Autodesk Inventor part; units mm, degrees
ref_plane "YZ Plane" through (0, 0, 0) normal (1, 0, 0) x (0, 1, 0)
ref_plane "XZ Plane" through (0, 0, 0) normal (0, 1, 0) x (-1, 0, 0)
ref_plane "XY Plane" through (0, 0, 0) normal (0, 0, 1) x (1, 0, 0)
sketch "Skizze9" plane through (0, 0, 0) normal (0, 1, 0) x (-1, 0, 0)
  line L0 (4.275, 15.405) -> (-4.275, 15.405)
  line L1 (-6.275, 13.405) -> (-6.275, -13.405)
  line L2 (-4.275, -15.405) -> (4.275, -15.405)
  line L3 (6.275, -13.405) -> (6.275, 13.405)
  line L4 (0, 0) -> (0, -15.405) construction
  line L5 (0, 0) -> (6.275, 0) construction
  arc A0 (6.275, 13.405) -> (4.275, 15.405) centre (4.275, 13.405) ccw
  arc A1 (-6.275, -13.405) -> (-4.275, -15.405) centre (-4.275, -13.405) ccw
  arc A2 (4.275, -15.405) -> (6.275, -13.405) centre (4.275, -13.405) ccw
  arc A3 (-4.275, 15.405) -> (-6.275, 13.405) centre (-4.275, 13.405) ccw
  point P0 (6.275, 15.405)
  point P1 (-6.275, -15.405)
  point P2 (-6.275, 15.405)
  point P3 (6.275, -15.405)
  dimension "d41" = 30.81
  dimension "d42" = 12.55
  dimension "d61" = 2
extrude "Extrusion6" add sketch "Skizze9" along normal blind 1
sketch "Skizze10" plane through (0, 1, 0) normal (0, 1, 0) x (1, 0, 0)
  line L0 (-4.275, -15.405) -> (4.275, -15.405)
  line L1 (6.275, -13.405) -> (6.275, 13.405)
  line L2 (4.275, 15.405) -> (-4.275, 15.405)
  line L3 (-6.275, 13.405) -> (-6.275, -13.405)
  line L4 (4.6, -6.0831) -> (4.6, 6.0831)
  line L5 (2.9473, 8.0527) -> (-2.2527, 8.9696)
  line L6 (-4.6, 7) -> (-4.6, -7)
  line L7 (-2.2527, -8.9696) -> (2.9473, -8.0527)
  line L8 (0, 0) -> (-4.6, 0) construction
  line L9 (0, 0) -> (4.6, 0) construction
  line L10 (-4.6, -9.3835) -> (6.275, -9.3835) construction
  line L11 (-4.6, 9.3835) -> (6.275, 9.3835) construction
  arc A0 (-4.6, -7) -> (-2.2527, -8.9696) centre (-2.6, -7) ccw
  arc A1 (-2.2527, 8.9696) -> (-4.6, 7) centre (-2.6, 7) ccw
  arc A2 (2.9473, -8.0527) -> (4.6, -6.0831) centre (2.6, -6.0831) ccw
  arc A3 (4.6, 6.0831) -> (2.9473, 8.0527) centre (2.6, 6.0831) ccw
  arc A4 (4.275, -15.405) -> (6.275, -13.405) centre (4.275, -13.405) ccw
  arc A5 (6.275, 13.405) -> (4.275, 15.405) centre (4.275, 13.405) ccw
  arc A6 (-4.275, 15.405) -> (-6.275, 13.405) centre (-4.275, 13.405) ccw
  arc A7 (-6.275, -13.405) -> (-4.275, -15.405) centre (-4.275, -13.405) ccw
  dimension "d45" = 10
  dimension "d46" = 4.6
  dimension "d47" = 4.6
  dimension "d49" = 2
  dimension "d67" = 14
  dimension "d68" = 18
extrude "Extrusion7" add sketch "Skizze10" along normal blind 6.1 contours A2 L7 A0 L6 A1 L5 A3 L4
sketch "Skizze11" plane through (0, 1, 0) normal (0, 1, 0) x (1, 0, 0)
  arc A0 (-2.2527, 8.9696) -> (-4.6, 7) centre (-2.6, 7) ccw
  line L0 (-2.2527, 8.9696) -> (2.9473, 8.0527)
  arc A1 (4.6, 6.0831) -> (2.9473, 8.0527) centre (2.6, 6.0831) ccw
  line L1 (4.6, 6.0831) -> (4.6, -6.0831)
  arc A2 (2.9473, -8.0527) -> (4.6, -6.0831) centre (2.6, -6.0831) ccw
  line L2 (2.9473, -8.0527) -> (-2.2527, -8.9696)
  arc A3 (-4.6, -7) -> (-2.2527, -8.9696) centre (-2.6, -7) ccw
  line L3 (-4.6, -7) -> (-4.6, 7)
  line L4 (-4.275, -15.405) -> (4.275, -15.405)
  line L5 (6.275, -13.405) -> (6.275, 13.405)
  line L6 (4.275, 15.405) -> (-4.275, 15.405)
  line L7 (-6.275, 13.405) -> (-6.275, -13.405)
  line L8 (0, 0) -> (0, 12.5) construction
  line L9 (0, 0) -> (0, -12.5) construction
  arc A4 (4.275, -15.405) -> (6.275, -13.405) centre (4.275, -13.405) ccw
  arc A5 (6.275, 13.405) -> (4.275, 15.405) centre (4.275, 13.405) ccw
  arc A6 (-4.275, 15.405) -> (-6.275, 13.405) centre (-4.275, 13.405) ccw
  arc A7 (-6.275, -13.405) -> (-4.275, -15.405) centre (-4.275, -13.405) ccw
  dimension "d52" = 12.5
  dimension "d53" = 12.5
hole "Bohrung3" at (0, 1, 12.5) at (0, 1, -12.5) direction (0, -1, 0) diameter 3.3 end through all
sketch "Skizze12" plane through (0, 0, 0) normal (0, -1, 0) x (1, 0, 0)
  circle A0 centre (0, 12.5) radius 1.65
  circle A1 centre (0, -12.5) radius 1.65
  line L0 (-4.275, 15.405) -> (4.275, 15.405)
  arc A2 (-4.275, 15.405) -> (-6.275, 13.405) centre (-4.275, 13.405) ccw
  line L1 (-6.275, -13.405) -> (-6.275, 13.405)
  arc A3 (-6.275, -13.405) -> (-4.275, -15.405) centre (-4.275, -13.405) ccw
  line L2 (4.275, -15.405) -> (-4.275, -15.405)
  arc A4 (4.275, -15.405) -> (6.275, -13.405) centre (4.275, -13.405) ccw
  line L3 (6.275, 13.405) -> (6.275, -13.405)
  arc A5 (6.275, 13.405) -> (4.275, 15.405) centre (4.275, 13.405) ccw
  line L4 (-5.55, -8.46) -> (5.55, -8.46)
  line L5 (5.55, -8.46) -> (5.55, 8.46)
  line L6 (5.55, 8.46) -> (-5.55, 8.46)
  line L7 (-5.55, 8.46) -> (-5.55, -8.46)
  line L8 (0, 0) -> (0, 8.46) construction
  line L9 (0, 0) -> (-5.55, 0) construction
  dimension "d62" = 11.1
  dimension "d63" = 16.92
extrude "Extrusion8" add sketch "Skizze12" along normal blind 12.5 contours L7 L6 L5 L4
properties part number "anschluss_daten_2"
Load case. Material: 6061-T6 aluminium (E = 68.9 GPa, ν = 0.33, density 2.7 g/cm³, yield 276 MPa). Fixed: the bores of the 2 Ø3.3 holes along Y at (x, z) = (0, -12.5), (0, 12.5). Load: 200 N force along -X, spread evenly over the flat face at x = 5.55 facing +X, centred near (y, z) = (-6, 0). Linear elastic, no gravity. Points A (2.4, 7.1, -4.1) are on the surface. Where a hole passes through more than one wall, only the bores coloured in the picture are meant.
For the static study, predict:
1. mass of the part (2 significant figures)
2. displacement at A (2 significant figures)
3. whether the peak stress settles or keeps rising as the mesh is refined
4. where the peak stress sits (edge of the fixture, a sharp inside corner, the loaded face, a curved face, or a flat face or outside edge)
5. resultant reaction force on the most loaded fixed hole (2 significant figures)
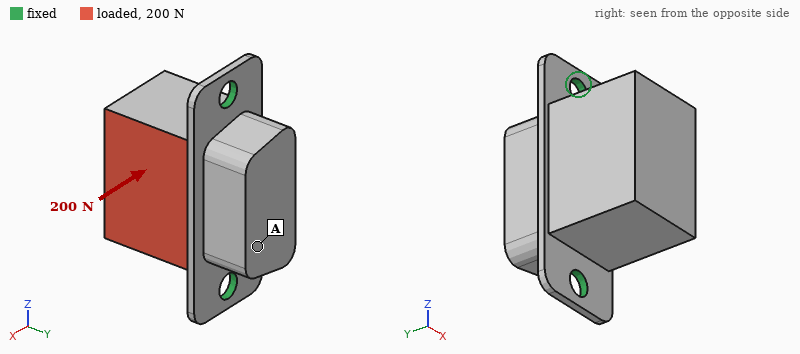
9.9 g
0.067 mm
keeps rising
edge of the fixture
100 N
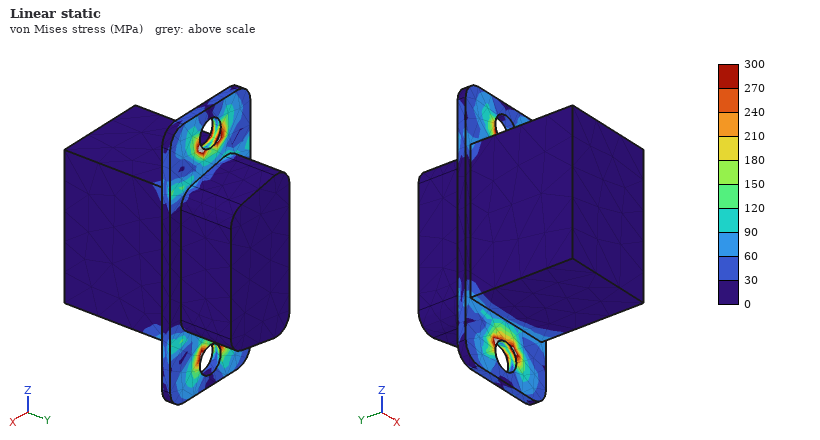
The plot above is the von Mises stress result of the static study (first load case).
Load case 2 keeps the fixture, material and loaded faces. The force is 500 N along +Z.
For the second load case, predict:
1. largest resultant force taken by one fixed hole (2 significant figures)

320 N
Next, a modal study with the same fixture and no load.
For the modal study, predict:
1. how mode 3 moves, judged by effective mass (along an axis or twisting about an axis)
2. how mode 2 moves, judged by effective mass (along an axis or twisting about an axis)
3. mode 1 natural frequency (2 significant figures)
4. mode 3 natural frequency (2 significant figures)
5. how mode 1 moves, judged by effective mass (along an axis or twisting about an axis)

along Z
along Y
2600 Hz
10 kHz
along X
